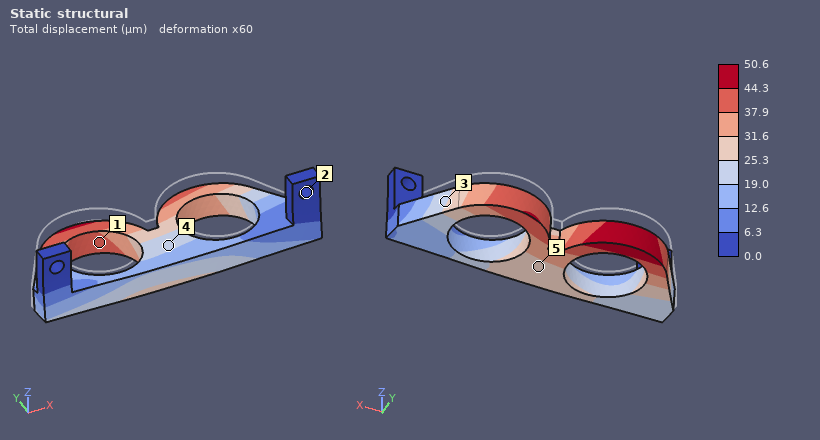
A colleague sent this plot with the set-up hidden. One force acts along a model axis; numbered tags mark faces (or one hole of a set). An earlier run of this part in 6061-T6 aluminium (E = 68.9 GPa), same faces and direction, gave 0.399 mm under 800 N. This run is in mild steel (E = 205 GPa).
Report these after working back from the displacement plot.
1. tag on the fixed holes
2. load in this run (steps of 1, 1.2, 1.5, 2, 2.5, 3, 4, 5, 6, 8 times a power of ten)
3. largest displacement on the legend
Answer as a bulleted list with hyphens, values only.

- 2
- 300 N
- 50.6 µm
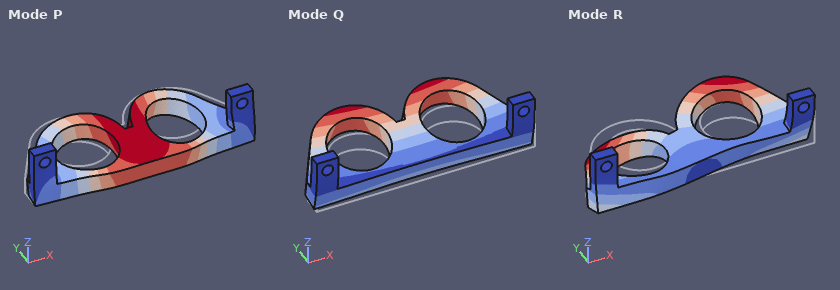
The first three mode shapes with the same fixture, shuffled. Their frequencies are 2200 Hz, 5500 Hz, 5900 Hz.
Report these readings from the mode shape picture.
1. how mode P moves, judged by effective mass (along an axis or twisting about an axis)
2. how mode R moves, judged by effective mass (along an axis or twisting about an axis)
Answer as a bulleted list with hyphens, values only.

- along Y
- along X
